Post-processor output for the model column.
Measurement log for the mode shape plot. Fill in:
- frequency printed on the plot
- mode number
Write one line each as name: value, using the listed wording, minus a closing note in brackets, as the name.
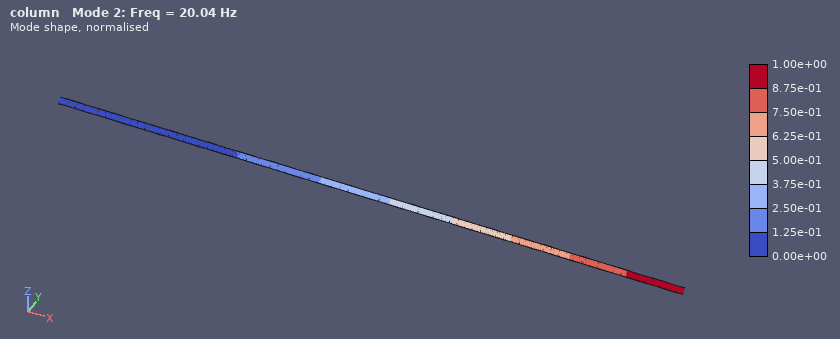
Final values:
frequency printed on the plot: 20.04 Hz
mode number: 2
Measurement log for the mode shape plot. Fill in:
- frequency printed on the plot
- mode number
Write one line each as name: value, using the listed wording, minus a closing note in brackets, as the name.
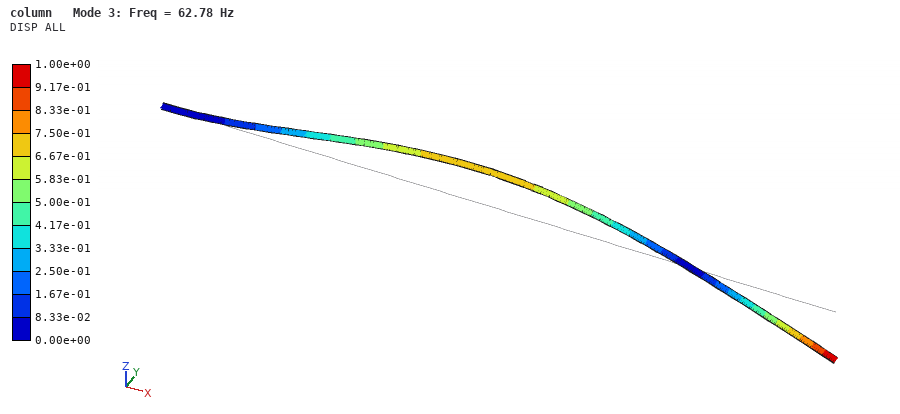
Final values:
frequency printed on the plot: 62.78 Hz
mode number: 3
